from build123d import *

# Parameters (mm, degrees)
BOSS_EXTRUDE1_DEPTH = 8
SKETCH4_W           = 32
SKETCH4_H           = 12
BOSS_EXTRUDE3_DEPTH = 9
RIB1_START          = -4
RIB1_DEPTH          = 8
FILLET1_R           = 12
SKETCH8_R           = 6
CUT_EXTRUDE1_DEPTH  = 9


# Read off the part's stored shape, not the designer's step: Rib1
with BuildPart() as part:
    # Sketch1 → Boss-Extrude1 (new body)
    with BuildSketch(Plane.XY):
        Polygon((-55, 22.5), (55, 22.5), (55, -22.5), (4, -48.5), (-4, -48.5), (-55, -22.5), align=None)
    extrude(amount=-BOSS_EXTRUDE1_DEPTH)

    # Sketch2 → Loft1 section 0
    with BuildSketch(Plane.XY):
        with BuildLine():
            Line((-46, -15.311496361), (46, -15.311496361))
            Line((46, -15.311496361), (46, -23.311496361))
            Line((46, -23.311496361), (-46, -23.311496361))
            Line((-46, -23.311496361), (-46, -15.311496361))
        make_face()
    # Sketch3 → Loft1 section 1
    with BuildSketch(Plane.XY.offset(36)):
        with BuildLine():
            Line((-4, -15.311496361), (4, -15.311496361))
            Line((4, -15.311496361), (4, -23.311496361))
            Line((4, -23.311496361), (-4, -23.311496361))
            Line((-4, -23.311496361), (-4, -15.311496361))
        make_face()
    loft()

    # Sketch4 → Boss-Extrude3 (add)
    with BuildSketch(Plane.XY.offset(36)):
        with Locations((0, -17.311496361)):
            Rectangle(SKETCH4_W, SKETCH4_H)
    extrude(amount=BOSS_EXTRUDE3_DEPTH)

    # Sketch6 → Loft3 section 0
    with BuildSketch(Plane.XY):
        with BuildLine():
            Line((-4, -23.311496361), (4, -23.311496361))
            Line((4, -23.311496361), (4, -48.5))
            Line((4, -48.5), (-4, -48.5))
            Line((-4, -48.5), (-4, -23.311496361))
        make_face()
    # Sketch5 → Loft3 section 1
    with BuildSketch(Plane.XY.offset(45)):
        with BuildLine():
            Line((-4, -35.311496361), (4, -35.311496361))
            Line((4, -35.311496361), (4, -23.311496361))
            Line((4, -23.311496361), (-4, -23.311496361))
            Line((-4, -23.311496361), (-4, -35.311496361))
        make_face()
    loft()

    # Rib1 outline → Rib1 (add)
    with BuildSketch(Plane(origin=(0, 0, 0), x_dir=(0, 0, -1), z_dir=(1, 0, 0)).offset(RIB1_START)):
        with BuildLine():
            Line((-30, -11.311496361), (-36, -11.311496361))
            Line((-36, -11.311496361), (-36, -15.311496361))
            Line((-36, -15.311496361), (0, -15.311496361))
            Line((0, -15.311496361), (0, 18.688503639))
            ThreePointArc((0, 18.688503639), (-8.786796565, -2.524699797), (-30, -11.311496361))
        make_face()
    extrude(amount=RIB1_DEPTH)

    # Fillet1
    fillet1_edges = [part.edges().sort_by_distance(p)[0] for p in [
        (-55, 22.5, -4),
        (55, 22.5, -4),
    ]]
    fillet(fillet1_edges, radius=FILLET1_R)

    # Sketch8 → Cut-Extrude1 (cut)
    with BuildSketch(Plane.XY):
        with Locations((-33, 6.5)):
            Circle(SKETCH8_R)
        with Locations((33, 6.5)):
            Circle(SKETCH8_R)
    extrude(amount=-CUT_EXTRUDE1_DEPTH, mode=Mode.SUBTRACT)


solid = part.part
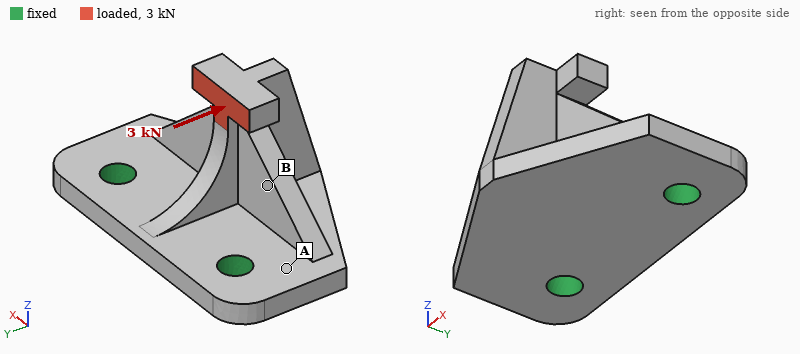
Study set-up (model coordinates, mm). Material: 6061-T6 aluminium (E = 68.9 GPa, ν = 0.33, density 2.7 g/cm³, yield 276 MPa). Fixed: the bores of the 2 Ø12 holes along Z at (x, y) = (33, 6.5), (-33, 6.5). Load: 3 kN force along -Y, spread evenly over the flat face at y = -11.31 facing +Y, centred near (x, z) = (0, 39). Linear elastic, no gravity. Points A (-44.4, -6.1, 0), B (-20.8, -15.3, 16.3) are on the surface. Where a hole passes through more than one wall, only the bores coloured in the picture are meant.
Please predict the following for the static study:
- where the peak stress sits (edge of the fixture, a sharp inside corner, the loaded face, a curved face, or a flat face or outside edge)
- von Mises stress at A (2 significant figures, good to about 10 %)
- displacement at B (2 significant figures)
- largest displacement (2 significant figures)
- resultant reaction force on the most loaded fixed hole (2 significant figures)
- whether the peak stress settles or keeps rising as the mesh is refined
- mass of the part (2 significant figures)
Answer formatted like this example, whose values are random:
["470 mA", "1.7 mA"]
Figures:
["edge of the fixture", "63 MPa", "0.16 mm", "0.45 mm", "1.5 kN", "keeps rising", "210 g"]
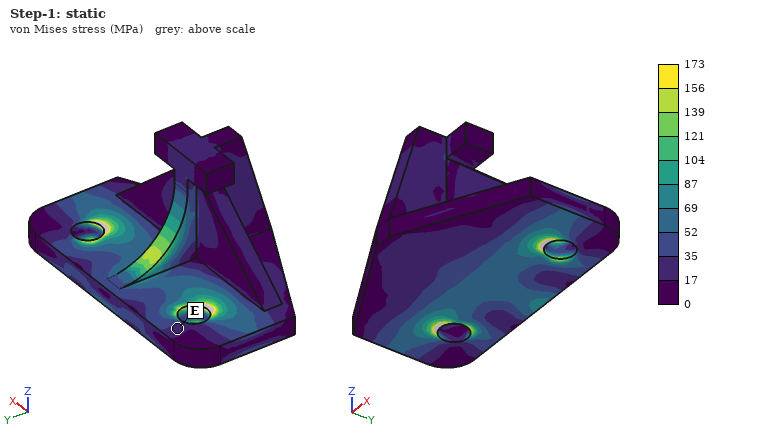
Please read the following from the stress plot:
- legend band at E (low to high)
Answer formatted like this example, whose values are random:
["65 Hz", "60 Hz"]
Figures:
["17 to 35 MPa"]
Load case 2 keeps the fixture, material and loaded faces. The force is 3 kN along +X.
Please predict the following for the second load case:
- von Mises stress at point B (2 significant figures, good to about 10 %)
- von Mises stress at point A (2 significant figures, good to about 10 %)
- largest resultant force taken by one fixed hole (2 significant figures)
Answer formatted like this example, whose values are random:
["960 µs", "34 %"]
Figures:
["32 MPa", "21 MPa", "2.5 kN"]
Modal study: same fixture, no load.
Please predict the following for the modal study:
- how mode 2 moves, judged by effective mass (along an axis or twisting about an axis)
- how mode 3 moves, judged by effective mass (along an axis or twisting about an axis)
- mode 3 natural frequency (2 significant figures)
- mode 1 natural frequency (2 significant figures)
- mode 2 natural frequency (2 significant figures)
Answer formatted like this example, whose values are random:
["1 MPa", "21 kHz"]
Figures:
["along X", "along Z", "6200 Hz", "2000 Hz", "4900 Hz"]
